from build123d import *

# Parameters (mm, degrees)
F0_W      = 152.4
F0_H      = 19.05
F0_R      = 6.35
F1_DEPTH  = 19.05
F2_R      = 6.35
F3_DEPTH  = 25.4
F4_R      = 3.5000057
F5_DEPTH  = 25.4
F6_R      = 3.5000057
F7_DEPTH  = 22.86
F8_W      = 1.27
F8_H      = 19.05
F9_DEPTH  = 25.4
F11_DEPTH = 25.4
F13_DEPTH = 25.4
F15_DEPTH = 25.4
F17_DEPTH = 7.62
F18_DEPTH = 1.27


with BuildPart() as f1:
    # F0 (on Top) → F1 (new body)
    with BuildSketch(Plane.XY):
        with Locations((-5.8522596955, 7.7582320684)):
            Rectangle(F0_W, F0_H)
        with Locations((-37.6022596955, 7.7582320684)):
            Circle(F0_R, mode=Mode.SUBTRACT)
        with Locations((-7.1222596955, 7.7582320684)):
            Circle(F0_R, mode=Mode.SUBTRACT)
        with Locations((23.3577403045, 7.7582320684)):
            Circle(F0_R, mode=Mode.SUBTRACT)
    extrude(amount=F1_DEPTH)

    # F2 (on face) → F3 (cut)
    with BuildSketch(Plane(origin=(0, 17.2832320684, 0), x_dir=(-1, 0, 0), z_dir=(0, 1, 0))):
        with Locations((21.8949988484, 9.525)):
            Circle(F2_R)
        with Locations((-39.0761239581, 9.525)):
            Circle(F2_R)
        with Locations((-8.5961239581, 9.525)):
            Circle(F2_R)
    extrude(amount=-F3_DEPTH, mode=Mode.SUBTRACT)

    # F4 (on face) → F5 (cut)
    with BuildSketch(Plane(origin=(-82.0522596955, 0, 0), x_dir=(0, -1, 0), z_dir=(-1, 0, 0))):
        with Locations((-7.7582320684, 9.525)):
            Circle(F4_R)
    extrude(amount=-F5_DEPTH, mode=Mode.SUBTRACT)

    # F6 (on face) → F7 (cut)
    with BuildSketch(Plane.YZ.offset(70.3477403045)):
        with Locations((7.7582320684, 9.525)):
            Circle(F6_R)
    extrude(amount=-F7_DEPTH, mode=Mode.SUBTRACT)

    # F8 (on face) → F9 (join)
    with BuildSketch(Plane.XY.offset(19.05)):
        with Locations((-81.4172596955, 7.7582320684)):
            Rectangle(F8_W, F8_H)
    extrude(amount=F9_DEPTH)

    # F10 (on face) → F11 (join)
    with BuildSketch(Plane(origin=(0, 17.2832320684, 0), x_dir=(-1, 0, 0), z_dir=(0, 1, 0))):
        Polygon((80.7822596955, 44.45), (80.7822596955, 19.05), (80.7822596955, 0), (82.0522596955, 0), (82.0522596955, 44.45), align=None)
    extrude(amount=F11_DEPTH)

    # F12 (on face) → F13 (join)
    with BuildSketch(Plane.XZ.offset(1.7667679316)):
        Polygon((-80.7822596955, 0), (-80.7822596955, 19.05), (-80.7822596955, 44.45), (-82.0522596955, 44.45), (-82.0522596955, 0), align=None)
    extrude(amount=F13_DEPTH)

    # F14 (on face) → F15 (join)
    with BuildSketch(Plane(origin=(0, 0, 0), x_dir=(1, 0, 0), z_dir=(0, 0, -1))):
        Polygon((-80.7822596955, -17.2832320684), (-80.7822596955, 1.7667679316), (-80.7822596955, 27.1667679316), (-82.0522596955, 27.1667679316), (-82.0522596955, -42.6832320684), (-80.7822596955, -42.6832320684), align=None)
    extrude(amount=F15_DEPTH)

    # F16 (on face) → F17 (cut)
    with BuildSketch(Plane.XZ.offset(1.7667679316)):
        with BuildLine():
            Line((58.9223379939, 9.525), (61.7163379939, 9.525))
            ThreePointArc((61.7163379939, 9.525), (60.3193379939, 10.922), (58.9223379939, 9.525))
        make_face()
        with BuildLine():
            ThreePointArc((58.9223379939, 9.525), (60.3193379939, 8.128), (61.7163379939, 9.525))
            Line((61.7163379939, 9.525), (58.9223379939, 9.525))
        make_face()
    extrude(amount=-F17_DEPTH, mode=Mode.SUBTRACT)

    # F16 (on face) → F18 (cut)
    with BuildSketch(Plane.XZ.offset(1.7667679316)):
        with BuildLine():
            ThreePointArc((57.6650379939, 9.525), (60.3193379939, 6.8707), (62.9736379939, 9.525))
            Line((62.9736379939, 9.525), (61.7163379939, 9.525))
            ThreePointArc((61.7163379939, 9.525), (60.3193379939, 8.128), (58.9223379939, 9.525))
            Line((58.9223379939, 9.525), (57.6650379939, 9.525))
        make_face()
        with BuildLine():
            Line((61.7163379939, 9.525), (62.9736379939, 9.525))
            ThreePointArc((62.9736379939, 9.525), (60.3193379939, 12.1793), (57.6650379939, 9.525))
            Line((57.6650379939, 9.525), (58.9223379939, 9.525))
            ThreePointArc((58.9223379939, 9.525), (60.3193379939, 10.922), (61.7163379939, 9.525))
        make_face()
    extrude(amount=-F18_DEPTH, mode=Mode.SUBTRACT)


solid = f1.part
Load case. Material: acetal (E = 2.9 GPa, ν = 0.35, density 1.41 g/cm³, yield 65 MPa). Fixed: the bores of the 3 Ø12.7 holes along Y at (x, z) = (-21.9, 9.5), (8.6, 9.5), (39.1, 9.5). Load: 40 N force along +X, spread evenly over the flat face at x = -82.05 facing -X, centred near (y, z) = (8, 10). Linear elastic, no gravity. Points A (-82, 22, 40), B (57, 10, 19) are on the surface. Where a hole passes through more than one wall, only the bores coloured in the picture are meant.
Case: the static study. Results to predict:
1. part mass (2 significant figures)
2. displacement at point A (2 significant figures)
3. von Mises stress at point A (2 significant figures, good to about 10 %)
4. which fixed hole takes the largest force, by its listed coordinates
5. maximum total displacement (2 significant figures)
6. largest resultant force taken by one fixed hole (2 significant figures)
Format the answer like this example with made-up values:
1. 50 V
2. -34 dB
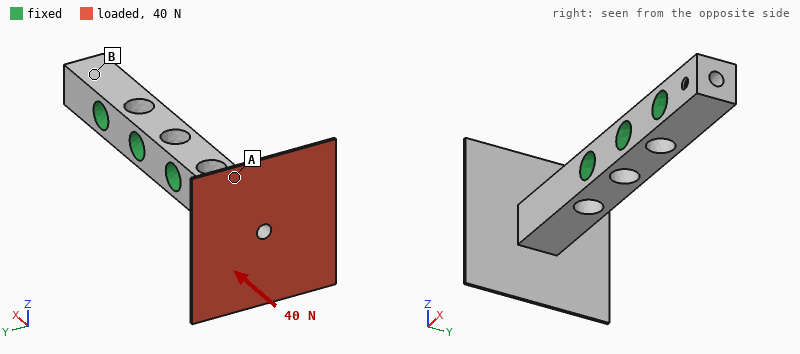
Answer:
1. 63 g
2. 0.95 mm
3. 3.2 MPa
4. (-21.9, 9.5)
5. 2.0 mm
6. 40 N
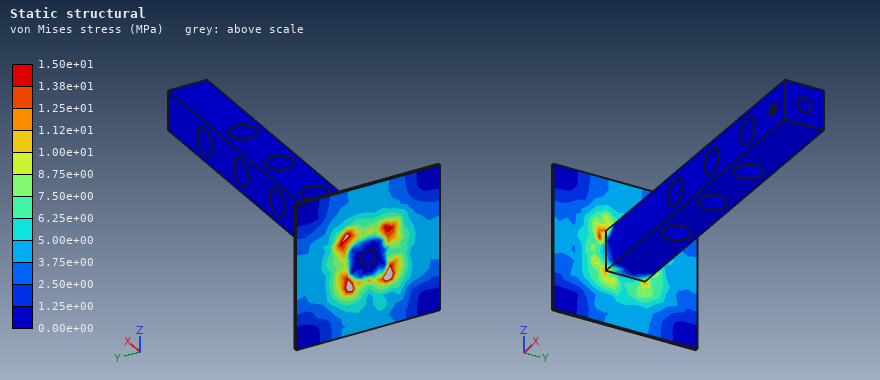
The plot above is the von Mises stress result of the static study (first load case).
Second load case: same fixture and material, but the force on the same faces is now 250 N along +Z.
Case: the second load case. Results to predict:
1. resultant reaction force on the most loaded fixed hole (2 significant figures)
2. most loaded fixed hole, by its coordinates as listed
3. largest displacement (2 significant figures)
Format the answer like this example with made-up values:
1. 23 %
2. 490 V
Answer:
1. 260 N
2. (-21.9, 9.5)
3. 1.8 mm
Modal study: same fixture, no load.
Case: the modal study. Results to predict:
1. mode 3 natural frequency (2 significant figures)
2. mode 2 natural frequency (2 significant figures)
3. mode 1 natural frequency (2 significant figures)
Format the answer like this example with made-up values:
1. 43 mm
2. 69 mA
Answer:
1. 340 Hz
2. 320 Hz
3. 320 Hz
